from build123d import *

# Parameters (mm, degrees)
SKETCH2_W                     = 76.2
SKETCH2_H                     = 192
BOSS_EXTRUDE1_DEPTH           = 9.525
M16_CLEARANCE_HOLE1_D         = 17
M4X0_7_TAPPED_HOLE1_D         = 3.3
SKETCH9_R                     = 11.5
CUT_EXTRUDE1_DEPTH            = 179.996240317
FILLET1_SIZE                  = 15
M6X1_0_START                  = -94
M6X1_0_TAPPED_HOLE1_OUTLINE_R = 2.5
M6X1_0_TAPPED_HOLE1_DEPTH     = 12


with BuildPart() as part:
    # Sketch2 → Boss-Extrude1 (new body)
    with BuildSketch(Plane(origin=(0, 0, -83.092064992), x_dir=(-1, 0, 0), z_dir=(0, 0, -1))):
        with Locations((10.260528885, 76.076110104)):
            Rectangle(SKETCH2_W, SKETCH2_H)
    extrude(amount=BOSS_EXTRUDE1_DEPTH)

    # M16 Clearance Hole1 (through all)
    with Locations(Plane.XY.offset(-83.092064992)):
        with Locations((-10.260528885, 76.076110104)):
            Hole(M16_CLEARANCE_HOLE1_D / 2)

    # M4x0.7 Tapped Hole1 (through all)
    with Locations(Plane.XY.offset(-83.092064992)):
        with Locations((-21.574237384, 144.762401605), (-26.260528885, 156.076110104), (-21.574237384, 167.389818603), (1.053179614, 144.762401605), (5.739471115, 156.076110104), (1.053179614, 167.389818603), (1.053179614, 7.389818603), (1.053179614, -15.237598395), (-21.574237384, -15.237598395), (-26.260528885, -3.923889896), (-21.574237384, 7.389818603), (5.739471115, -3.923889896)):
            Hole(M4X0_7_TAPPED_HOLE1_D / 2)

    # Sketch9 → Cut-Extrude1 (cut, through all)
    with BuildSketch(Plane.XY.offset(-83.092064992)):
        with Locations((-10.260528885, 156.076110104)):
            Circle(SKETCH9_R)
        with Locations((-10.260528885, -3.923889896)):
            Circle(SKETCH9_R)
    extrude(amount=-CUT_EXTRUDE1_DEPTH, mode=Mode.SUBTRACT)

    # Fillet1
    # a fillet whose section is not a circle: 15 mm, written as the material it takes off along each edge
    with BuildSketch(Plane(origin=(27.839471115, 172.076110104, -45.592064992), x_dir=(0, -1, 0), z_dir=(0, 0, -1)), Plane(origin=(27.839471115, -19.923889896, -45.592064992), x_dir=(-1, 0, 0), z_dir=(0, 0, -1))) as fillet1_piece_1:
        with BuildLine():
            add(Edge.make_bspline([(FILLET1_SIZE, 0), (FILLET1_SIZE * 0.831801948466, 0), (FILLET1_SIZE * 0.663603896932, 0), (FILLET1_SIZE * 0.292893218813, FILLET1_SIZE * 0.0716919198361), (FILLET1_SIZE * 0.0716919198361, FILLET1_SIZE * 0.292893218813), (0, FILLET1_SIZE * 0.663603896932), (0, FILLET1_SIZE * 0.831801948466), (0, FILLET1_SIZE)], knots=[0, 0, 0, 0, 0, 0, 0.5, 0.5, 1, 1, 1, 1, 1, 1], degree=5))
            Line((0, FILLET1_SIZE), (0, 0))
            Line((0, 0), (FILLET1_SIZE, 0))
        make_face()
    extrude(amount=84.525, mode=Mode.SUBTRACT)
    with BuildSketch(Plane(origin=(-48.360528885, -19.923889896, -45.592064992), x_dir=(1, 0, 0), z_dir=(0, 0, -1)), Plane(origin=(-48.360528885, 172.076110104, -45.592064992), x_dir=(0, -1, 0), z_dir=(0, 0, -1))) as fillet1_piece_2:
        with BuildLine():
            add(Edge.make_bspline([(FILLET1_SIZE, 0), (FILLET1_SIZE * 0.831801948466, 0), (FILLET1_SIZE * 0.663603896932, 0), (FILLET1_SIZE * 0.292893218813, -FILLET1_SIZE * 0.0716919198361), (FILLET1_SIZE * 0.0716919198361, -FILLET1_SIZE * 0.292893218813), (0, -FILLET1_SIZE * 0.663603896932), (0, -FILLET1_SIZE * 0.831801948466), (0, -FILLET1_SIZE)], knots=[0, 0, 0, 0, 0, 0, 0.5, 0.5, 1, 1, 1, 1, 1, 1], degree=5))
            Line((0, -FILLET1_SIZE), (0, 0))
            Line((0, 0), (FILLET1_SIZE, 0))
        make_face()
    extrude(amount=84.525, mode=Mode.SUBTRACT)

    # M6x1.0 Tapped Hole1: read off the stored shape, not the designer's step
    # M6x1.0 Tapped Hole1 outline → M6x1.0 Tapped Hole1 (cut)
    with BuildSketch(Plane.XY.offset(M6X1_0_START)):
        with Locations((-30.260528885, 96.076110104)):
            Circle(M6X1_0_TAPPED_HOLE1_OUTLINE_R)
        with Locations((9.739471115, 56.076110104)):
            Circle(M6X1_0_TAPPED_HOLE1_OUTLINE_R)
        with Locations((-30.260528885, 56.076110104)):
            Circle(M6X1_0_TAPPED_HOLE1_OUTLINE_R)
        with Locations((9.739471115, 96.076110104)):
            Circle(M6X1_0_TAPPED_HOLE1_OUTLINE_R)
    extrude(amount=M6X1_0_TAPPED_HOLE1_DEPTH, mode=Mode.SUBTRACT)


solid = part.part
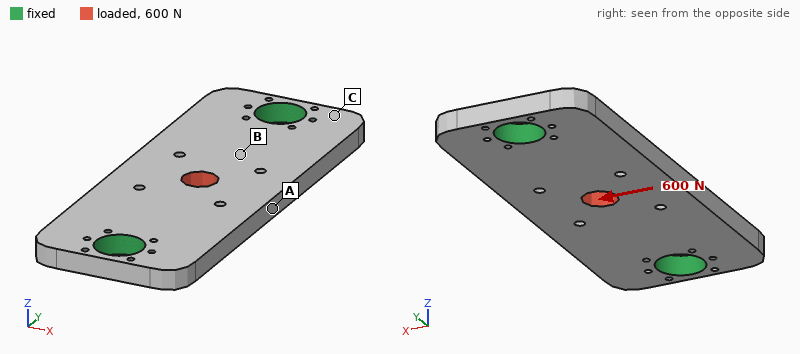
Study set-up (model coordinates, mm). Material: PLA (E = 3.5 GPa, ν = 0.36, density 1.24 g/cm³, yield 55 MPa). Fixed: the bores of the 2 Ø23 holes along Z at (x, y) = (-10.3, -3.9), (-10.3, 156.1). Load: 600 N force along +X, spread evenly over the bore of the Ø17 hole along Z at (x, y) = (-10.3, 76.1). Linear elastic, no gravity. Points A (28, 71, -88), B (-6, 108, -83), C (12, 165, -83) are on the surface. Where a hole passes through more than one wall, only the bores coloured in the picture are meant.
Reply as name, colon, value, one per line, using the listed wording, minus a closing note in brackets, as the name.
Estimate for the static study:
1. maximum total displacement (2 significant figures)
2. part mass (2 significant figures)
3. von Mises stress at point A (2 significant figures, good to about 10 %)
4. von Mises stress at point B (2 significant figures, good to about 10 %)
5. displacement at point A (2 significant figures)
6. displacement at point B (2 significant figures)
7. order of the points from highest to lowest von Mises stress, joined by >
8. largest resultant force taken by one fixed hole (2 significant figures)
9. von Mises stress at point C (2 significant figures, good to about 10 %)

maximum total displacement: 51 µm
part mass: 160 g
von Mises stress at point A: 2.0 MPa
von Mises stress at point B: 0.94 MPa
displacement at point A: 44 µm
displacement at point B: 32 µm
order of the points from highest to lowest von Mises stress, joined by >: A > B > C
largest resultant force taken by one fixed hole: 300 N
von Mises stress at point C: 0.38 MPa
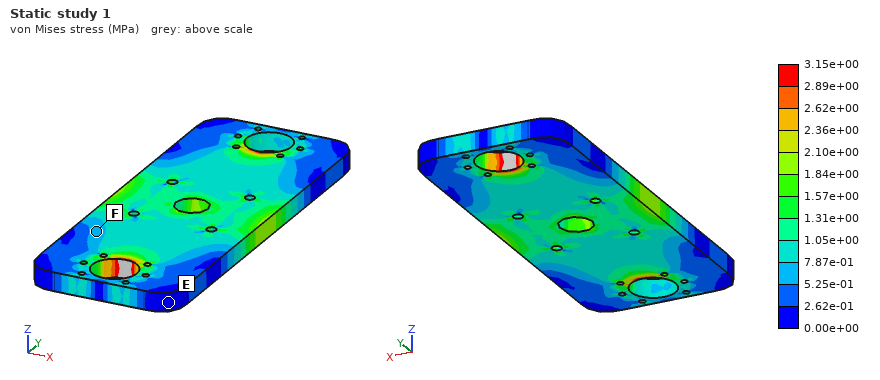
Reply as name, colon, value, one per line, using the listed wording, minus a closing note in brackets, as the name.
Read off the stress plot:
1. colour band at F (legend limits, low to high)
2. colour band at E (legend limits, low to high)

colour band at F: 5.25e-01 to 7.87e-01 MPa
colour band at E: 0.00e+00 to 2.62e-01 MPa
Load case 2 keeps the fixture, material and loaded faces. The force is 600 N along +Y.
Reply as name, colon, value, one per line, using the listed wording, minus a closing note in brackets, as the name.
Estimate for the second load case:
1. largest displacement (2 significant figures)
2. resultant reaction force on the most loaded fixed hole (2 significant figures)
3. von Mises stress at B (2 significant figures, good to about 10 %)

largest displacement: 15 µm
resultant reaction force on the most loaded fixed hole: 300 N
von Mises stress at B: 0.79 MPa
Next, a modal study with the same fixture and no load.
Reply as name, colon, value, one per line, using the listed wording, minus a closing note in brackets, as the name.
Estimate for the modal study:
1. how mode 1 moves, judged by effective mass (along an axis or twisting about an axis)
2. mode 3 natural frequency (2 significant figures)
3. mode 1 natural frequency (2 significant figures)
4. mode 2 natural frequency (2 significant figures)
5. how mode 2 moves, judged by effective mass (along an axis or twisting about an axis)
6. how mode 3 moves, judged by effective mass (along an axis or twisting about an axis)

how mode 1 moves, judged by effective mass: along Z
mode 3 natural frequency: 1800 Hz
mode 1 natural frequency: 710 Hz
mode 2 natural frequency: 900 Hz
how mode 2 moves, judged by effective mass: twisting about Y
how mode 3 moves, judged by effective mass: twisting about X
